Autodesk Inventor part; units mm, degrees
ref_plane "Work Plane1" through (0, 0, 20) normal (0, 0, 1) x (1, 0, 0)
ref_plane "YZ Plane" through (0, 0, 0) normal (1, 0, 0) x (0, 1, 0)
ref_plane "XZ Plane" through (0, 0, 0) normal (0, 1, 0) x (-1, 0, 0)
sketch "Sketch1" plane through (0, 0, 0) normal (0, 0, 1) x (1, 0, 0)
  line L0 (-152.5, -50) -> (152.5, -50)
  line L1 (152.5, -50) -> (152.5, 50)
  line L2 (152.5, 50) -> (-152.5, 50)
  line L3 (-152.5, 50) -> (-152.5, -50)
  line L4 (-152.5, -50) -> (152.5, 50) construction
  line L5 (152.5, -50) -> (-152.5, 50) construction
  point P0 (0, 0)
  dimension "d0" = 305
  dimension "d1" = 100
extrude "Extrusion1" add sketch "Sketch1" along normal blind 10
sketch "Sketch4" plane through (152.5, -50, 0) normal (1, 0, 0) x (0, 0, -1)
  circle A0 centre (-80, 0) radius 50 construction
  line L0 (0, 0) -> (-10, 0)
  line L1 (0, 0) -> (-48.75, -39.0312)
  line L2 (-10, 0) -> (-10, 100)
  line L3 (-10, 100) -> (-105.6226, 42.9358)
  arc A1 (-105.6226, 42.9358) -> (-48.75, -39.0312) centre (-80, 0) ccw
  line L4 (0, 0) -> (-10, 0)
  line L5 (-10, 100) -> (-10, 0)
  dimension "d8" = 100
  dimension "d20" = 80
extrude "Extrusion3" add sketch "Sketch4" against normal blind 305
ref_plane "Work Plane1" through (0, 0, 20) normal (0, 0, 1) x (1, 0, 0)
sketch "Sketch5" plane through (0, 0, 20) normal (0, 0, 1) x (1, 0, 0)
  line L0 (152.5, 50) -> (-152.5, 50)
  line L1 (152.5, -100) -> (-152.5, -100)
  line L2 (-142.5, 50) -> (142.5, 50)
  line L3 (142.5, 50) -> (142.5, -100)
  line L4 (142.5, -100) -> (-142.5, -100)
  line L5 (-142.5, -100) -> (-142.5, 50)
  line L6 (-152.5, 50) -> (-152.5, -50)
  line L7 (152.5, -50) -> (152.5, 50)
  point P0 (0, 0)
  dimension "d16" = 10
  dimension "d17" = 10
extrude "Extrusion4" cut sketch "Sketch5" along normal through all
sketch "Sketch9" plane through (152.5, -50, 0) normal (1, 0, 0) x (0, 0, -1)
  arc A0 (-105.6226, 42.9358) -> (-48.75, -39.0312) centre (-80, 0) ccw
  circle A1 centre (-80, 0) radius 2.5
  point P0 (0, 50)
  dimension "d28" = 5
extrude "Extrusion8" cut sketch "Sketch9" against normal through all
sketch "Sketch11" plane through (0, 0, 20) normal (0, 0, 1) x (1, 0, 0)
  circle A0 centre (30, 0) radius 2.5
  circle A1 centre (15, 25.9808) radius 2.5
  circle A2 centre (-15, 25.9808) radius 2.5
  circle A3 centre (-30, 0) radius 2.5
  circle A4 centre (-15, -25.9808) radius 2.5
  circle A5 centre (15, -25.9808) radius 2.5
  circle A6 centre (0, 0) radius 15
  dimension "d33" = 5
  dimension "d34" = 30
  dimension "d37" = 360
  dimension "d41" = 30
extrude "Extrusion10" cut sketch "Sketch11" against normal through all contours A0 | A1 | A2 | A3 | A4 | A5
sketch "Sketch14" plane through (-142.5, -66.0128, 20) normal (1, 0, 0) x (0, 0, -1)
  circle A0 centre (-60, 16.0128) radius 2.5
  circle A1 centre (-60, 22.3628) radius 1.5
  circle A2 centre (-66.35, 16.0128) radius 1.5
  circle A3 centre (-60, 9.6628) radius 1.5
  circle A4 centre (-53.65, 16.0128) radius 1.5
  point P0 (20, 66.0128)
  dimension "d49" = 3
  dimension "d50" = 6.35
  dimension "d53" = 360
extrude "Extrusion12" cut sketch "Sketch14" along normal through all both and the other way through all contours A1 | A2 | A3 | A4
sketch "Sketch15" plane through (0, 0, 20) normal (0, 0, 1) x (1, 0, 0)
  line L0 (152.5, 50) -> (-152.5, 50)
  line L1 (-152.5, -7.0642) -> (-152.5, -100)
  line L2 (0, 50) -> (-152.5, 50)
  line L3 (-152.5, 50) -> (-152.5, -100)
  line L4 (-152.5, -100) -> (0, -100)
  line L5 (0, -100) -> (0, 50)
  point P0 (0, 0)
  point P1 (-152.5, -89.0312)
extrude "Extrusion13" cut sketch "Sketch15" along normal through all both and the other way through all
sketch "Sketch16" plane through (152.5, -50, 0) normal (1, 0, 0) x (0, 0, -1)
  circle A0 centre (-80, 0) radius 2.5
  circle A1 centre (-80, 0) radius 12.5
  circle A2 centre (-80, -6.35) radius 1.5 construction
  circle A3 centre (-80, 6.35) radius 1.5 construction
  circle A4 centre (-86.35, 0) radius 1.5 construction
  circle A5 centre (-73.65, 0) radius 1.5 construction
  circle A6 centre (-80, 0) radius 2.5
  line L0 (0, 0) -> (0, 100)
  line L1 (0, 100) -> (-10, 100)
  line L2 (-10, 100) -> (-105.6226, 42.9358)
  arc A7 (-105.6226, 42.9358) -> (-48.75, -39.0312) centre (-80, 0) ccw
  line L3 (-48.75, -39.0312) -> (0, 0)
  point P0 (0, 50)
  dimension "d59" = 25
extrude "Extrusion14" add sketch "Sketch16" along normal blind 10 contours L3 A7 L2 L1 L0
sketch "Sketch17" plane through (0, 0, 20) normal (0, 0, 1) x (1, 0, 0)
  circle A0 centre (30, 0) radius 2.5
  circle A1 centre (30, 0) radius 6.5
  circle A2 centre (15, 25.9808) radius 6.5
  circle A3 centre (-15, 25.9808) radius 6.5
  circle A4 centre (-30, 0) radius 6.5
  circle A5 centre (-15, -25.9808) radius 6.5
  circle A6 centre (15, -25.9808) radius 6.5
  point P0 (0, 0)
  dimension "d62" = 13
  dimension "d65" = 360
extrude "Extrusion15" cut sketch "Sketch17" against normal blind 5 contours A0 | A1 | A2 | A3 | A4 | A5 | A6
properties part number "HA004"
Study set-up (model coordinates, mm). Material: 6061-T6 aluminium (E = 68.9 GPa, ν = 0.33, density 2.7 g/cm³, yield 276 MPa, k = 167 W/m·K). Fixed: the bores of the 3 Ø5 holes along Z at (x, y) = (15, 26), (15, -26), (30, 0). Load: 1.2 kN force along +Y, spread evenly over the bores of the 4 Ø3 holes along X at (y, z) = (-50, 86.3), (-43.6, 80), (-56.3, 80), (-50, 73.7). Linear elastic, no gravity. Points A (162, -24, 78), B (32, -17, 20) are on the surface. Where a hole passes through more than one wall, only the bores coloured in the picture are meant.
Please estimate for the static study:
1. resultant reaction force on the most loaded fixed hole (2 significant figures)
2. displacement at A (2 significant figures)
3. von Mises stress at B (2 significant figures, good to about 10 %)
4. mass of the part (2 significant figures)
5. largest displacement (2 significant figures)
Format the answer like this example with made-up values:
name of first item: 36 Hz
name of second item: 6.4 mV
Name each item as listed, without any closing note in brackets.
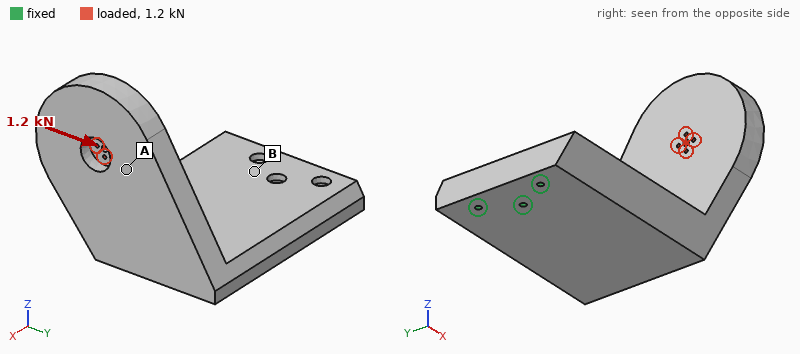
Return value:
resultant reaction force on the most loaded fixed hole: 2.9 kN
displacement at A: 0.12 mm
von Mises stress at B: 12 MPa
mass of the part: 1.5 kg
largest displacement: 0.22 mm
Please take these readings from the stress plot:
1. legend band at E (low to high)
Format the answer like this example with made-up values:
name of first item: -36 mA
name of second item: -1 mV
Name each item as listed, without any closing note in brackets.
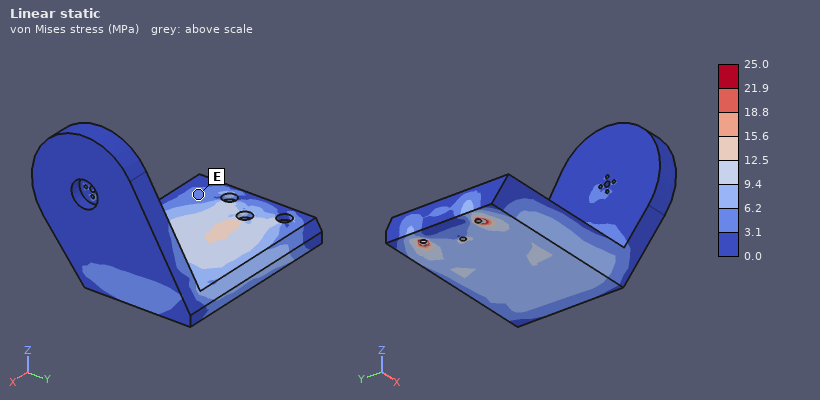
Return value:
legend band at E: 3.1 to 6.2 MPa
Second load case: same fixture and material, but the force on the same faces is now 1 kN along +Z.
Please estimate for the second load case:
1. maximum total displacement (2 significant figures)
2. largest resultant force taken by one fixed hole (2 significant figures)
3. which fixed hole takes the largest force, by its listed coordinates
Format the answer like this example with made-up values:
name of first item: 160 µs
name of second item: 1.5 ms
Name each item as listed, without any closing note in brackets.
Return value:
maximum total displacement: 0.35 mm
largest resultant force taken by one fixed hole: 3.3 kN
which fixed hole takes the largest force, by its listed coordinates: (30, 0)
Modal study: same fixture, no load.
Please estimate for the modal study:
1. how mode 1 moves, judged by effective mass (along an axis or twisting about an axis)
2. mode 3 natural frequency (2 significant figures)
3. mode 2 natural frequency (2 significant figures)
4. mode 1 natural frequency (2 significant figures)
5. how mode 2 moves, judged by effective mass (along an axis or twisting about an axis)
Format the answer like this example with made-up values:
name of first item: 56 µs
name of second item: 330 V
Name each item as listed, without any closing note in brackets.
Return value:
how mode 1 moves, judged by effective mass: along Z
mode 3 natural frequency: 1000 Hz
mode 2 natural frequency: 610 Hz
mode 1 natural frequency: 330 Hz
how mode 2 moves, judged by effective mass: along Y
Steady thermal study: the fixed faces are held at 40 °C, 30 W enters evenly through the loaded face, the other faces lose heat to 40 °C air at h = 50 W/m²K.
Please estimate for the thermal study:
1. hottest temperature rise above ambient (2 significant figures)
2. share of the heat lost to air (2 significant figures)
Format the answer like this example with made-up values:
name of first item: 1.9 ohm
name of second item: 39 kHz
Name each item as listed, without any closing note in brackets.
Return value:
hottest temperature rise above ambient: 14 K
share of the heat lost to air: 59 %
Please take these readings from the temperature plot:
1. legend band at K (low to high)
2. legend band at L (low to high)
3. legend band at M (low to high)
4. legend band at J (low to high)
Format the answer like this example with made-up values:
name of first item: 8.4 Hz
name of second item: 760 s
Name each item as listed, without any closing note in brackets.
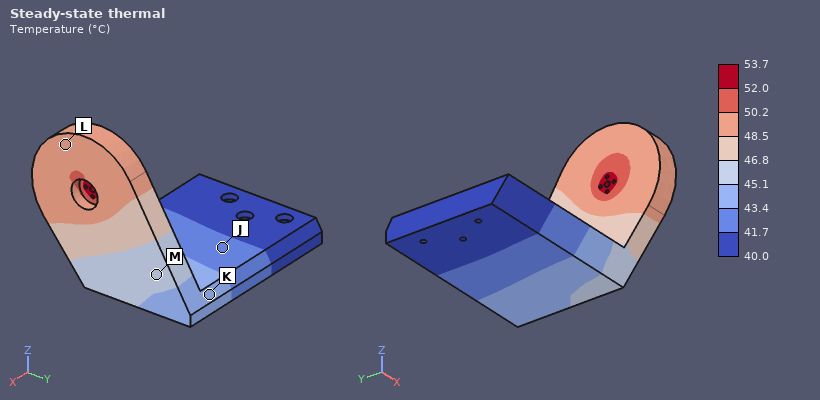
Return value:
legend band at K: 43.4 to 45.1 °C
legend band at L: 48.5 to 50.2 °C
legend band at M: 45.1 to 46.8 °C
legend band at J: 41.7 to 43.4 °C
